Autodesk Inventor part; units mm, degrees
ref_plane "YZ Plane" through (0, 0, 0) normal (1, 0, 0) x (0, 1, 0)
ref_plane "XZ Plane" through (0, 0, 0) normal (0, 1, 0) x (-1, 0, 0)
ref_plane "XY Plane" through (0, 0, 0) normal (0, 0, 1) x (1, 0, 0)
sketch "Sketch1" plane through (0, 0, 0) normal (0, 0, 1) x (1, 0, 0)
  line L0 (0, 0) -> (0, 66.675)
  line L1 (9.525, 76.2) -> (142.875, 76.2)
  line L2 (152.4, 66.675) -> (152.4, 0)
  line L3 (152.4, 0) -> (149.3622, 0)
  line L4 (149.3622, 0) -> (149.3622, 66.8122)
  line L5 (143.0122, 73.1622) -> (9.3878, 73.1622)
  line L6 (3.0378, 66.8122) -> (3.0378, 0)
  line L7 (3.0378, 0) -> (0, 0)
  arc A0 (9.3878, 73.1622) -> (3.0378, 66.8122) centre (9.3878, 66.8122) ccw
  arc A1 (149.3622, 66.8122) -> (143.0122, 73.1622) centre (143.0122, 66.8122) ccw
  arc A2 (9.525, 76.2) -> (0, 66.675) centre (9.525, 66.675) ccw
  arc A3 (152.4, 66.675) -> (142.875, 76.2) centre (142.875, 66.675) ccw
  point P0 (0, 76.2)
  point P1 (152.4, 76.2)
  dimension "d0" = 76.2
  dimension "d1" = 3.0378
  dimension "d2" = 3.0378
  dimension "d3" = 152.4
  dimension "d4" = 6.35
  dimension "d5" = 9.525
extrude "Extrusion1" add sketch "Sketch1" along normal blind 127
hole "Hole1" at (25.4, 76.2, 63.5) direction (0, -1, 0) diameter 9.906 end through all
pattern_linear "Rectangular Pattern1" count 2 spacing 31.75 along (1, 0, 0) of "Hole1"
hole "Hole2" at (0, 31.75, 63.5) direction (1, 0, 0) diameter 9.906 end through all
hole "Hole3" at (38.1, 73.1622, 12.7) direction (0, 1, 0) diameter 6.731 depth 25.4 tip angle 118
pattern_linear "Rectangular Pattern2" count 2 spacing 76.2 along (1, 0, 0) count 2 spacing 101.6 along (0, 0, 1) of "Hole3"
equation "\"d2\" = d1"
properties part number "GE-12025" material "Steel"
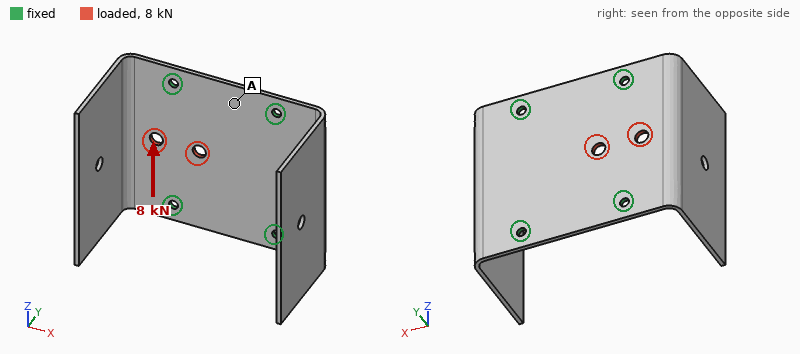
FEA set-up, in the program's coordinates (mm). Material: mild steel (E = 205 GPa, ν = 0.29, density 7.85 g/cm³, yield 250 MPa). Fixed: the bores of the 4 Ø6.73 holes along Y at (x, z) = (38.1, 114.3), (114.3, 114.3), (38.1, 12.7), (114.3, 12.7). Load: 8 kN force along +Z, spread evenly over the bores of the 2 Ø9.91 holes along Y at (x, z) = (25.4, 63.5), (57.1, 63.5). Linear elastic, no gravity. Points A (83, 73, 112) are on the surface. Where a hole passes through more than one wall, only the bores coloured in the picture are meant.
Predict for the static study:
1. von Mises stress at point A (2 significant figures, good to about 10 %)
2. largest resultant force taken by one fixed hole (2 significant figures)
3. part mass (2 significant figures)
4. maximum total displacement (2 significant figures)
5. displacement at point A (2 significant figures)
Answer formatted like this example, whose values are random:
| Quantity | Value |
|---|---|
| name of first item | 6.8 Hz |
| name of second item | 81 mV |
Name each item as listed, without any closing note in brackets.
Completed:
| Quantity | Value |
|---|---|
| von Mises stress at point A | 7.4 MPa |
| largest resultant force taken by one fixed hole | 3.2 kN |
| part mass | 870 g |
| maximum total displacement | 8.5 µm |
| displacement at point A | 2.8 µm |
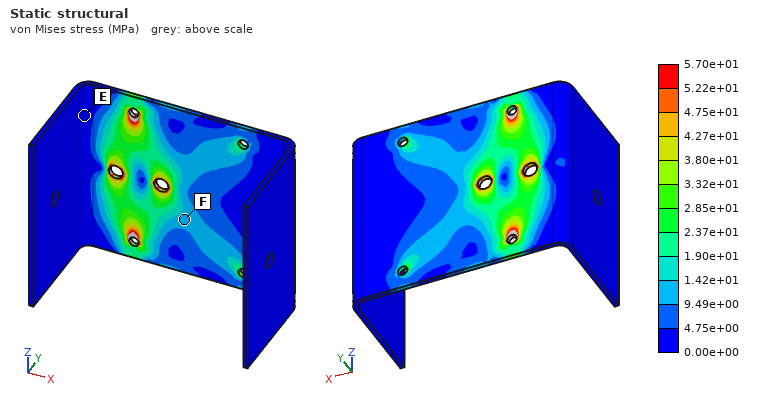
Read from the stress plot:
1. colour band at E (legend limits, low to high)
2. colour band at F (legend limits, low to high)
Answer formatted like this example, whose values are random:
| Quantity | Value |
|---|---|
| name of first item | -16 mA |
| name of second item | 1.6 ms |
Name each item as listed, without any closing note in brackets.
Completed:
| Quantity | Value |
|---|---|
| colour band at E | 0.00e+00 to 4.75e+00 MPa |
| colour band at F | 9.49e+00 to 1.42e+01 MPa |
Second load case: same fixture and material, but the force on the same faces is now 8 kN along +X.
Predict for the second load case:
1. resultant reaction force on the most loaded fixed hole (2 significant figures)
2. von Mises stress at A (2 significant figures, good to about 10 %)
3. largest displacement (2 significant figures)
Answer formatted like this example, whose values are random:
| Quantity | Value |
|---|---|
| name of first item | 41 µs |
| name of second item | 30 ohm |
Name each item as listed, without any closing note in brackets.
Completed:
| Quantity | Value |
|---|---|
| resultant reaction force on the most loaded fixed hole | 2.3 kN |
| von Mises stress at A | 12 MPa |
| largest displacement | 14 µm |
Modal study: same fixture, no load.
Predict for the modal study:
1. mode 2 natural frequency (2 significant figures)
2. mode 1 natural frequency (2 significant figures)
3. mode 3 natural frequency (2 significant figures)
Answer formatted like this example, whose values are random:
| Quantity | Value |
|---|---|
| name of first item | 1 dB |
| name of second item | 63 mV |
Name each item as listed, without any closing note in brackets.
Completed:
| Quantity | Value |
|---|---|
| mode 2 natural frequency | 250 Hz |
| mode 1 natural frequency | 250 Hz |
| mode 3 natural frequency | 520 Hz |
